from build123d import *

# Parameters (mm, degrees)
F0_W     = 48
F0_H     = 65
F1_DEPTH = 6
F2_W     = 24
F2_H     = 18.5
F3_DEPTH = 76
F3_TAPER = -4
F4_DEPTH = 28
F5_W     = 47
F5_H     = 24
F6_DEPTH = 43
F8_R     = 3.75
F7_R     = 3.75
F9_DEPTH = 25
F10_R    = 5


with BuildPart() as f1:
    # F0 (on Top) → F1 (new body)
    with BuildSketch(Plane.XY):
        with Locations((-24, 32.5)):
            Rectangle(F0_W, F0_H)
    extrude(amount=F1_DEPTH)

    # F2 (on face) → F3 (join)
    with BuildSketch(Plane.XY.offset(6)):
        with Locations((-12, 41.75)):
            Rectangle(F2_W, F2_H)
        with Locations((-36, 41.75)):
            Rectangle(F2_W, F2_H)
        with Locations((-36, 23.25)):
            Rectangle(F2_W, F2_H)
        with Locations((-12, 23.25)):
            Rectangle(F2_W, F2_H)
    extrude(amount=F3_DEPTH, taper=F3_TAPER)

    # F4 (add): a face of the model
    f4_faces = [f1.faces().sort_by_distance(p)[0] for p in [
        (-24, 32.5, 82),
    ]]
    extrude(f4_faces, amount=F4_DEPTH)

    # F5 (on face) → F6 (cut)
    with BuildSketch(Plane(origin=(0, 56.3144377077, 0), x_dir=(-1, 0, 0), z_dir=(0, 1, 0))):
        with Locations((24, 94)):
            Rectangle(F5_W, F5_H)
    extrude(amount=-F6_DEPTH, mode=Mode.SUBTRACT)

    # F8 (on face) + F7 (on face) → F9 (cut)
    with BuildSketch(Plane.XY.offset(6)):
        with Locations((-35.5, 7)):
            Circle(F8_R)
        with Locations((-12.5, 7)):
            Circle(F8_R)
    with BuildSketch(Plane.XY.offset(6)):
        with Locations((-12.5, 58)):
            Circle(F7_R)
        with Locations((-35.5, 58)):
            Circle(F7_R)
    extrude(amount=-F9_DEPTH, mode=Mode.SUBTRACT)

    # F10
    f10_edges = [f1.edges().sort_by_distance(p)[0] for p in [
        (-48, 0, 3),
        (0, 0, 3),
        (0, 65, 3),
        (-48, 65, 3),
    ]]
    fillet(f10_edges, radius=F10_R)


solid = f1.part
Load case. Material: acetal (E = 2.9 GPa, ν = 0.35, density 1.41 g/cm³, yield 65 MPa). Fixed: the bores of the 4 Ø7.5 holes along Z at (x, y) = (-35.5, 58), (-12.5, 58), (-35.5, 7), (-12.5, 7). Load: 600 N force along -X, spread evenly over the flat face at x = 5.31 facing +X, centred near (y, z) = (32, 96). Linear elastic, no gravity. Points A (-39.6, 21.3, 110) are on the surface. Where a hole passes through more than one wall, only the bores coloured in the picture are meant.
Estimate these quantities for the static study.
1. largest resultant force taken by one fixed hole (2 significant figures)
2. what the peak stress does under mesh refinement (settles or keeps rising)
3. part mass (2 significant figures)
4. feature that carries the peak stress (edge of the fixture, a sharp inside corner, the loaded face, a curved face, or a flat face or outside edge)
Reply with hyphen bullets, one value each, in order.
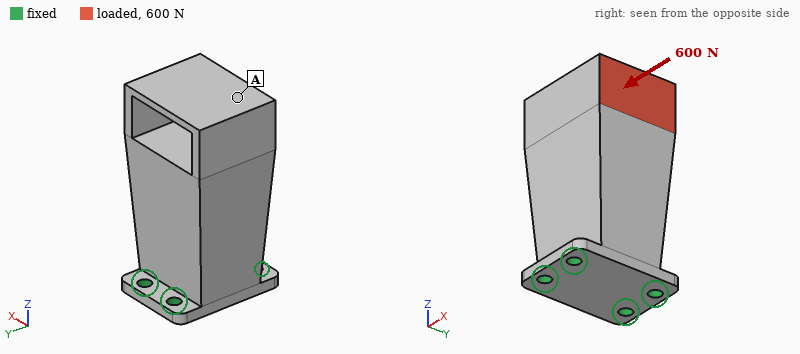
- 1.1 kN
- keeps rising
- 310 g
- edge of the fixture
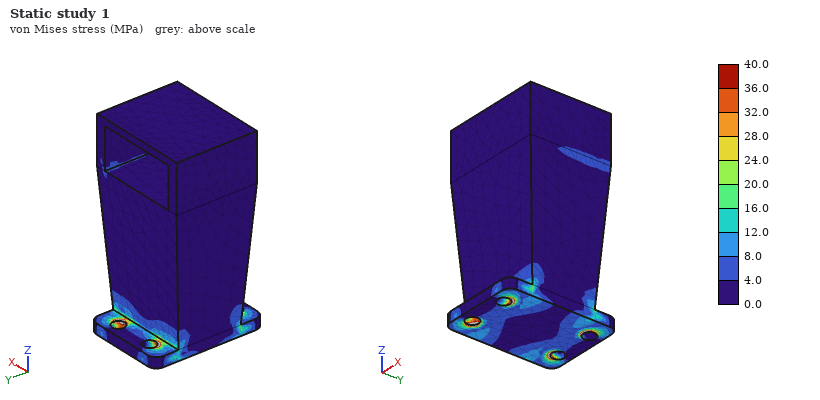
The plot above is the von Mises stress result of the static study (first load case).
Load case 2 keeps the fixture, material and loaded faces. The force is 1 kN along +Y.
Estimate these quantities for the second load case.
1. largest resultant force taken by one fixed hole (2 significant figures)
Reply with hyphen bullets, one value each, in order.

- 1.3 kN
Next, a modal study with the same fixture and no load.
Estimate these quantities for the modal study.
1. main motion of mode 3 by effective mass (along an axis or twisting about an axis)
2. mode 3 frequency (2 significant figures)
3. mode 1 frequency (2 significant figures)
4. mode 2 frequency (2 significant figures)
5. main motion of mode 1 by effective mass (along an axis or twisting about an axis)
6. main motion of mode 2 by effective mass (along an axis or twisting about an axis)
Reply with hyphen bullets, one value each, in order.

- twisting about Z
- 1500 Hz
- 350 Hz
- 510 Hz
- along X
- along Y
